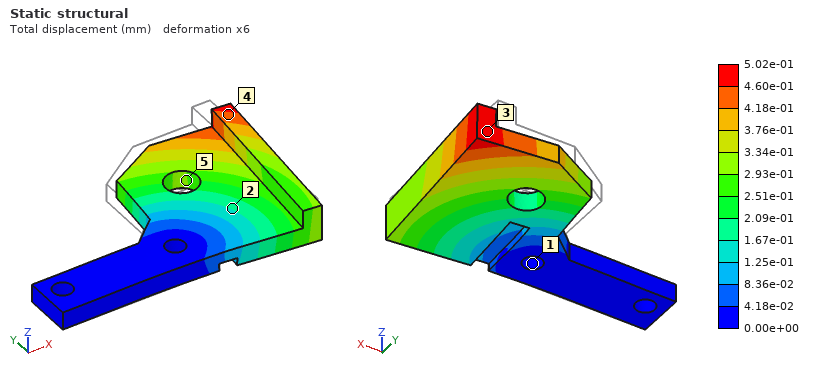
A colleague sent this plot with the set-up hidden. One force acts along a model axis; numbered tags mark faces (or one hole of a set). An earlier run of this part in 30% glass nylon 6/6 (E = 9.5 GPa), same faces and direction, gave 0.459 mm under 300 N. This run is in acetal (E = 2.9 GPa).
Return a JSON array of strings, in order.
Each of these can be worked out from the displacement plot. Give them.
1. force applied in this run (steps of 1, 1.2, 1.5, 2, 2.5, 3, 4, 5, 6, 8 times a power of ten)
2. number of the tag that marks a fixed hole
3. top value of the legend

["100 N", "1", "5.02e-01 mm"]
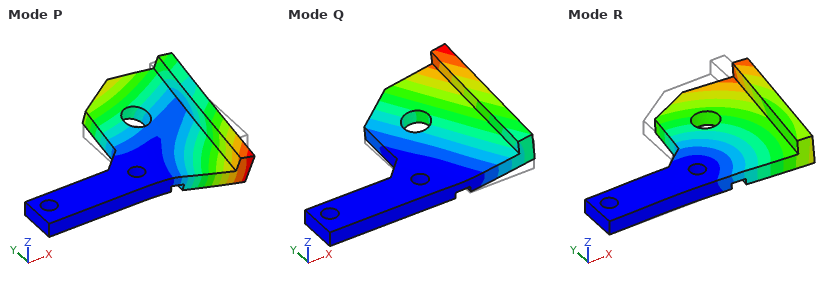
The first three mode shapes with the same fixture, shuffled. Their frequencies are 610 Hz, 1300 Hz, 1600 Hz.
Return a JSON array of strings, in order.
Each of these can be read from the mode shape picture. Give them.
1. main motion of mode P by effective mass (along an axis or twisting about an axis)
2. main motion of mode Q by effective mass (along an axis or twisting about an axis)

["twisting about X", "along Z"]
